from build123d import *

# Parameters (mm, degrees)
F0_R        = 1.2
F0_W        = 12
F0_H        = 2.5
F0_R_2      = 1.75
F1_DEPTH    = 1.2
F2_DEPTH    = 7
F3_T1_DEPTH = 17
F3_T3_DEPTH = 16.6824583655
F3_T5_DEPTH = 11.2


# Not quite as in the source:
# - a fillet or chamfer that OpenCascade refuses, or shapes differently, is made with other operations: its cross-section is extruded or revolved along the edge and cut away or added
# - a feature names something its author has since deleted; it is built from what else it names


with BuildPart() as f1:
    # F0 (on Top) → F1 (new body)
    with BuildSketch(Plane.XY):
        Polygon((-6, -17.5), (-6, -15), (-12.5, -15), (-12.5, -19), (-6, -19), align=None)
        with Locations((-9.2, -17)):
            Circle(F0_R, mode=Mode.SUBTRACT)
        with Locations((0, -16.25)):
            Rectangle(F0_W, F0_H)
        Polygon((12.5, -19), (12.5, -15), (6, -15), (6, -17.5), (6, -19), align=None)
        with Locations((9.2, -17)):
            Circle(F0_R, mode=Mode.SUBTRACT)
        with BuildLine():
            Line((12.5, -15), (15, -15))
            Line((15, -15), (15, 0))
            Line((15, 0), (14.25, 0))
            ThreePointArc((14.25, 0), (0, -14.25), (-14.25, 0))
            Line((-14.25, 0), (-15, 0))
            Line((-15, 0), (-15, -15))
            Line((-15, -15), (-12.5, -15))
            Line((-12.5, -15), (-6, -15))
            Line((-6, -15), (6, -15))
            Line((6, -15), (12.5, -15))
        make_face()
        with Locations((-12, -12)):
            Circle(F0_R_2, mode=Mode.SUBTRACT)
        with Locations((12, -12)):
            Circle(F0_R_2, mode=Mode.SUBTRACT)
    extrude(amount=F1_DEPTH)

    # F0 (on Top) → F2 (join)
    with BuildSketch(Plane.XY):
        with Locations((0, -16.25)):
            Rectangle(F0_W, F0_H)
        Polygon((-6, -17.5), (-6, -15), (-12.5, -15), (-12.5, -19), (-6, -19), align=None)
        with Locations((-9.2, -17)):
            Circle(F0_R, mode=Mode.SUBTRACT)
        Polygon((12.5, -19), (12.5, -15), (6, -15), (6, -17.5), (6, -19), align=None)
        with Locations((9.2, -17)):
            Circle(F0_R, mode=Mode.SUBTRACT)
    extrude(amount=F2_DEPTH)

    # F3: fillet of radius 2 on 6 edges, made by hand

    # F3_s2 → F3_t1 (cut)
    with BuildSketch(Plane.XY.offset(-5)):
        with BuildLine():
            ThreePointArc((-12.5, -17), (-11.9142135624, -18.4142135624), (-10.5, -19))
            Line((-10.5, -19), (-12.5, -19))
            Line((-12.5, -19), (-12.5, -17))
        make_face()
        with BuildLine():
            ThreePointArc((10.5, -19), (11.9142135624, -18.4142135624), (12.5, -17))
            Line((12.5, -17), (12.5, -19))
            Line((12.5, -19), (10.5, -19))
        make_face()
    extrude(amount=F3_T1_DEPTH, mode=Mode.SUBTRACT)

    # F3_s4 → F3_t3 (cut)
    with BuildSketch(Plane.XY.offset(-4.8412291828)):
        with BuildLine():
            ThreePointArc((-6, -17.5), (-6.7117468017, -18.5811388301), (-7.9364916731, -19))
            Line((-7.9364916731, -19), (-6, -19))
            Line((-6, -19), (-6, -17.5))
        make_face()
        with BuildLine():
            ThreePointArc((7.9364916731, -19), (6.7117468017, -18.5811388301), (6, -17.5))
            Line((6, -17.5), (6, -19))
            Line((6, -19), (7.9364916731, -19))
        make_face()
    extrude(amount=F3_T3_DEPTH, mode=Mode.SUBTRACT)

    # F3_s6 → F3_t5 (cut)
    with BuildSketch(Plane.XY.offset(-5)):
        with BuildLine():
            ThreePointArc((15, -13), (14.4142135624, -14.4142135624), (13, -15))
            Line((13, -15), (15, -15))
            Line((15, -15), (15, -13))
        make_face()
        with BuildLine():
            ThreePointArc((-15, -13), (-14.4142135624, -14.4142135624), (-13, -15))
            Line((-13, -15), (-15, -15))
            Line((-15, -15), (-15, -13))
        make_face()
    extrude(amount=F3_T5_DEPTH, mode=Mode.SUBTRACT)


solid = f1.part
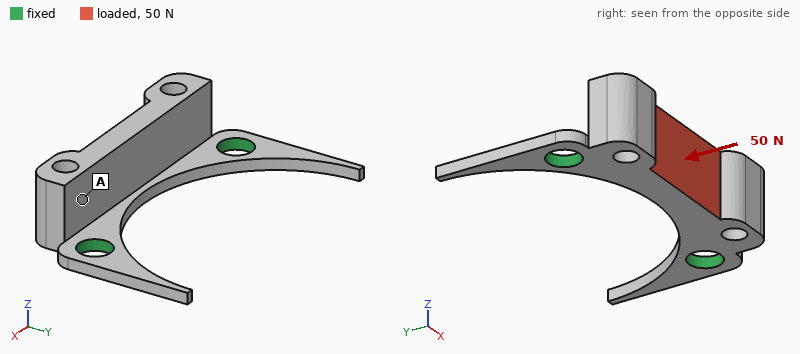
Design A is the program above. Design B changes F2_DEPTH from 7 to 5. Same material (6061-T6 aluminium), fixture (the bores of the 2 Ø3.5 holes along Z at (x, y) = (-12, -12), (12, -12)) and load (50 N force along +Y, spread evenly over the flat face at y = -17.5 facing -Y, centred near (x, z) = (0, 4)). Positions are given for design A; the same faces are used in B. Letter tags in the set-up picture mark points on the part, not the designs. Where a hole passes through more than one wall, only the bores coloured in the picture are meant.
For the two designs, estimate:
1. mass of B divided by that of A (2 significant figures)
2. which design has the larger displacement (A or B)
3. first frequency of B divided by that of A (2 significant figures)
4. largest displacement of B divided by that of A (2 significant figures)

0.78
A
1.4
0.59
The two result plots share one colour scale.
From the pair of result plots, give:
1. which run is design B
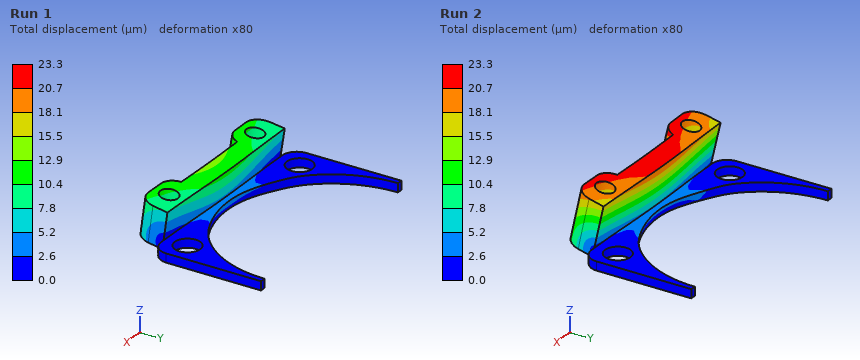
Run 1
